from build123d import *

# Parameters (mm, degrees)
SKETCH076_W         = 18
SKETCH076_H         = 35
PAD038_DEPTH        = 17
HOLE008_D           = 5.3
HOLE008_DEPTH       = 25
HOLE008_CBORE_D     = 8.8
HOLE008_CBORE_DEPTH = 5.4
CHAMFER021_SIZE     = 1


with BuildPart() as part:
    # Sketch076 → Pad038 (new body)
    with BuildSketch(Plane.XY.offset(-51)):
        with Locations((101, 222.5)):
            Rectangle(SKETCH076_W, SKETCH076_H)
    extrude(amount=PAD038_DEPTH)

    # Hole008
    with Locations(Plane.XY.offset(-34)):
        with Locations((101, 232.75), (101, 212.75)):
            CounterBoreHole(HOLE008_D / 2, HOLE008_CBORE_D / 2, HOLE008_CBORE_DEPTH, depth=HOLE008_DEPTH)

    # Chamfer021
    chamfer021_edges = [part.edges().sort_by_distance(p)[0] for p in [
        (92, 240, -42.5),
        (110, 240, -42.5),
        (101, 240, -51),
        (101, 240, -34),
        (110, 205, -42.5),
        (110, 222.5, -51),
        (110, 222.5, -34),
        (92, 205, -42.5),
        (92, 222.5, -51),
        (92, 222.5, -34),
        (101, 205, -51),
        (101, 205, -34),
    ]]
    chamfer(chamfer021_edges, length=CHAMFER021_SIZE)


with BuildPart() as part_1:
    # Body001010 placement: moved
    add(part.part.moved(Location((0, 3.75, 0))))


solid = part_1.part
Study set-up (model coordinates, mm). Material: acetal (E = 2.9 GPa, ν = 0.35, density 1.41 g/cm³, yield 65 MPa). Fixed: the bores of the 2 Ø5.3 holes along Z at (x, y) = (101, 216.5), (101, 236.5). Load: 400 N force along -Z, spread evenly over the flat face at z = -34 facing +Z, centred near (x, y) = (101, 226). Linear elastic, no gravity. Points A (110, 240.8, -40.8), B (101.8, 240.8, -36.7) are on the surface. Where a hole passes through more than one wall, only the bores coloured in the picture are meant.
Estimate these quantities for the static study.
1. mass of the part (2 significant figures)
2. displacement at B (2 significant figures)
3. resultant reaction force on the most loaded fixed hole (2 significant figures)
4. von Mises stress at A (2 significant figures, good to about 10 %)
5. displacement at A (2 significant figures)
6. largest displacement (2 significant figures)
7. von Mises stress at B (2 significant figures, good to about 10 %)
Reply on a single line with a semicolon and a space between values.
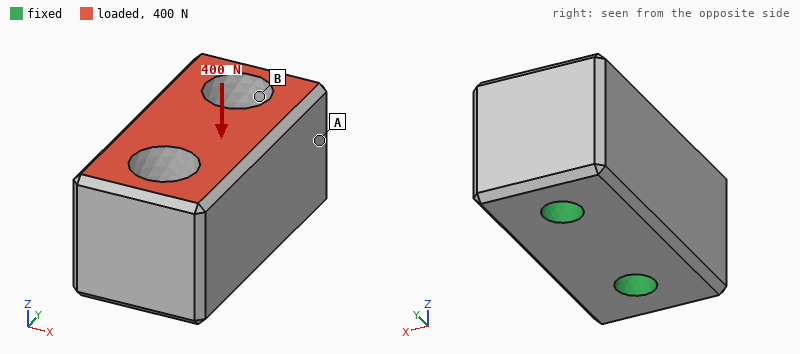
13 g; 3.4 µm; 210 N; 0.44 MPa; 3.5 µm; 6.1 µm; 1.4 MPa
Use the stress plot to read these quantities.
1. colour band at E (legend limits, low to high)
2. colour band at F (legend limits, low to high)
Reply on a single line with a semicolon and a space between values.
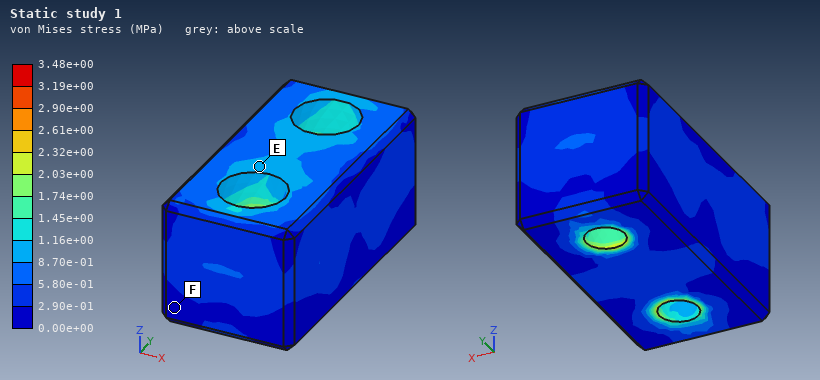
8.70e-01 to 1.16e+00 MPa; 0.00e+00 to 2.90e-01 MPa
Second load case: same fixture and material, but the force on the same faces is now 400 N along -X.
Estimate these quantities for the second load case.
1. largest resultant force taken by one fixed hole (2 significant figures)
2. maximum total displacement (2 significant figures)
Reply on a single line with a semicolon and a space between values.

210 N; 30 µm
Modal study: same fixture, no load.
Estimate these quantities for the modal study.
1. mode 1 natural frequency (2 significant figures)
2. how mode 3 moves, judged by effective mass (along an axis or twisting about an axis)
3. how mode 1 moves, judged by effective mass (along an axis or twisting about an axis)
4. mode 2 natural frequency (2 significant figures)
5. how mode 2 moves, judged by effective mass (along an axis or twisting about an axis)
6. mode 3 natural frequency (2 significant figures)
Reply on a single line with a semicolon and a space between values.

11 kHz; along Y; along X; 15 kHz; twisting about Z; 15 kHz
